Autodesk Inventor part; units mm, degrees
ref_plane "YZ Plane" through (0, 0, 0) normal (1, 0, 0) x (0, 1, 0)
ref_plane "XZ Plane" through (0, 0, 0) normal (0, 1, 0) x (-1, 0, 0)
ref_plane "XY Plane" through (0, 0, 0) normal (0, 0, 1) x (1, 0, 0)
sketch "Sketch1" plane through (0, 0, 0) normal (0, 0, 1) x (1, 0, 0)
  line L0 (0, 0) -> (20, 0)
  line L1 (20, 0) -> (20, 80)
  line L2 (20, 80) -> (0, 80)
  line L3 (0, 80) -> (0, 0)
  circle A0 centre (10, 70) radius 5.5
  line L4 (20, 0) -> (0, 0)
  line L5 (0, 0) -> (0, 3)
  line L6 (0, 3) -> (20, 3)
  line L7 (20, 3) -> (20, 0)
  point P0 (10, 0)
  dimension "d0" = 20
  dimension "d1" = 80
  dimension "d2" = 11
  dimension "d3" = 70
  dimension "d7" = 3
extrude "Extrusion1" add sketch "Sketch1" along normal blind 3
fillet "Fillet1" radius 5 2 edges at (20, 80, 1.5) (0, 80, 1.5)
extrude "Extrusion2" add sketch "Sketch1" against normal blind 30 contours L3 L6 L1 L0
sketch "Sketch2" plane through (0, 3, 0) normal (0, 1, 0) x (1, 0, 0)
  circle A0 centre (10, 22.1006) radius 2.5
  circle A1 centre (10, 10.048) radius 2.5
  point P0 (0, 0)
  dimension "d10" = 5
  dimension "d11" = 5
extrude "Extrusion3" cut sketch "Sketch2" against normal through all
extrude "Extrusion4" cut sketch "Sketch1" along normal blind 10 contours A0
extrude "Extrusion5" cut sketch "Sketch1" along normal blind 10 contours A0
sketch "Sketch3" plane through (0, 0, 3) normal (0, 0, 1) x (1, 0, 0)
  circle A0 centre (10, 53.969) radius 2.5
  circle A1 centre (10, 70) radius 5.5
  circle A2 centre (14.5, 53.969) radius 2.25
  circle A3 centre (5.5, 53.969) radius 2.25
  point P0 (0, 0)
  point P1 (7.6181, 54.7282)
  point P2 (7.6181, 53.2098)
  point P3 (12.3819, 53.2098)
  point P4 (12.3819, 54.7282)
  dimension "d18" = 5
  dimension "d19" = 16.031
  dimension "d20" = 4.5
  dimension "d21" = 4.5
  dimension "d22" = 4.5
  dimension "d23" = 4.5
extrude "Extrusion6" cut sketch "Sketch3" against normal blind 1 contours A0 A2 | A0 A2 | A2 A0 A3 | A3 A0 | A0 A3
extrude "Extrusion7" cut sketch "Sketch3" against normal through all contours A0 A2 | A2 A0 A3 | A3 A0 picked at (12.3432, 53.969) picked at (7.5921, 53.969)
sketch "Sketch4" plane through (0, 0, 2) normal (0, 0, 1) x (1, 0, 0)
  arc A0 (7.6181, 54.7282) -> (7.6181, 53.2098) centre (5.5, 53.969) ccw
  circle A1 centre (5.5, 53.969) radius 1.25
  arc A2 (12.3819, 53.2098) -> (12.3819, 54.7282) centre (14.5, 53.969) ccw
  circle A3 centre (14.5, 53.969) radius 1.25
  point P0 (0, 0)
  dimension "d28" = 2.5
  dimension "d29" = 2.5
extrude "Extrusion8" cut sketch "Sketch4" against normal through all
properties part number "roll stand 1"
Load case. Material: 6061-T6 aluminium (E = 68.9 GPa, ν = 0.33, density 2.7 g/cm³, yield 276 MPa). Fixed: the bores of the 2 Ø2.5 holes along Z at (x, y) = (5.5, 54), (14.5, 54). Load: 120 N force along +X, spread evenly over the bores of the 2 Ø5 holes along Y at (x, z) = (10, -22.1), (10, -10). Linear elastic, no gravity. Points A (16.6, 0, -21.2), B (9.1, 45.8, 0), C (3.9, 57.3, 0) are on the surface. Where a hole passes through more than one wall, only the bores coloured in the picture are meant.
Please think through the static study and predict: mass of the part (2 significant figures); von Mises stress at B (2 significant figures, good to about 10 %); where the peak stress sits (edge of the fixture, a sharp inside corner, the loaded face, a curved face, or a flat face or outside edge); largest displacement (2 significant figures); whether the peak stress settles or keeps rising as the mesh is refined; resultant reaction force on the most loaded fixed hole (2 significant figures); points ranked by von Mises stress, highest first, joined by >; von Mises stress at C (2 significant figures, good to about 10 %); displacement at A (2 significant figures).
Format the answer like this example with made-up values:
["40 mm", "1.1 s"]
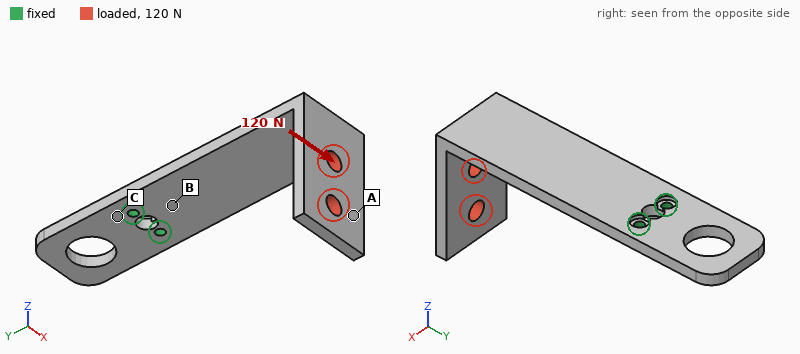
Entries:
["16 g", "73 MPa", "edge of the fixture", "0.86 mm", "keeps rising", "600 N", "B > C > A", "16 MPa", "0.63 mm"]
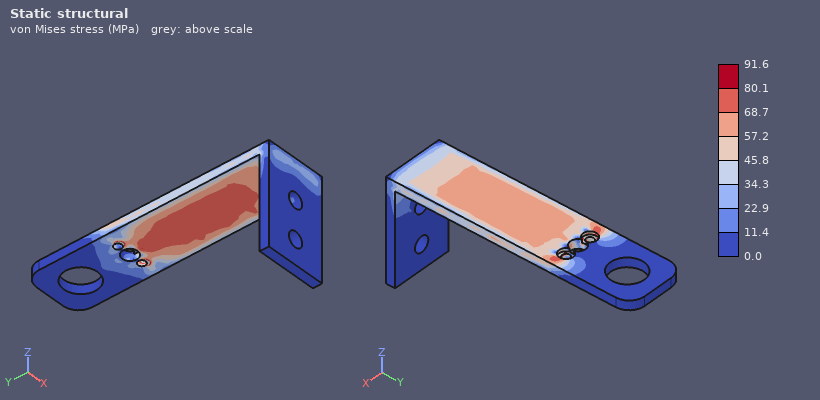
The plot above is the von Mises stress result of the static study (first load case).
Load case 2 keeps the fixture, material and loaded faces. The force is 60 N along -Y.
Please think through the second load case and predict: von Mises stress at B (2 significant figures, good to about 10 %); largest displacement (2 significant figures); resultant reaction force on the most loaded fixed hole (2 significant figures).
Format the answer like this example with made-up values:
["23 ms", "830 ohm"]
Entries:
["33 MPa", "0.87 mm", "30 N"]
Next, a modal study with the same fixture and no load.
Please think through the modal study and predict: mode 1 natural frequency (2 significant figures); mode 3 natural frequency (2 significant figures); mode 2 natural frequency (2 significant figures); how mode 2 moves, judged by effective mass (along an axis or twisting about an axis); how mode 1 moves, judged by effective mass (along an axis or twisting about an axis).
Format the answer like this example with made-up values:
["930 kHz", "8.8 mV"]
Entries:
["410 Hz", "1600 Hz", "1100 Hz", "along X", "along Z"]
